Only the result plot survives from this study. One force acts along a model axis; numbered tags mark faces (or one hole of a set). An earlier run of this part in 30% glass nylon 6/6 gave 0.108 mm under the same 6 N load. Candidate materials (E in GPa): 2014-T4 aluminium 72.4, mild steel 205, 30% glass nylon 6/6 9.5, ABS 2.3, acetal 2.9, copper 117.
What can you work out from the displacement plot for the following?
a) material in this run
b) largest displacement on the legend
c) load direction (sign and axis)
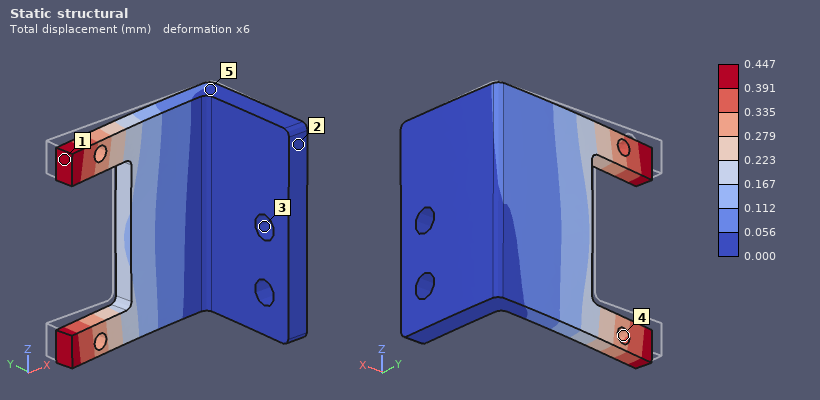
ABS
0.447 mm
-Y
